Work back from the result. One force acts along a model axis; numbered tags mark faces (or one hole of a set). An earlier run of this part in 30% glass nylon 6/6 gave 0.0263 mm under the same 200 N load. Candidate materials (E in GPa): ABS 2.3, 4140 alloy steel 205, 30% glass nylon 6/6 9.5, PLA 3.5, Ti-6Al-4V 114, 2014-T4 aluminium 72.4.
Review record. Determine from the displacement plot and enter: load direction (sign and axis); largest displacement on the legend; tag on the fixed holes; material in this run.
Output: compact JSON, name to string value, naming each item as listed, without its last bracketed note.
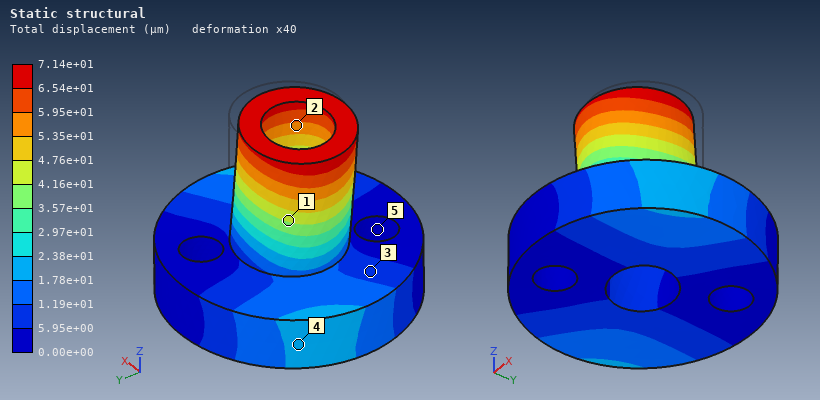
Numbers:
{"load direction": "-X", "largest displacement on the legend": "7.14e+01 µm", "tag on the fixed holes": "5", "material in this run": "PLA"}
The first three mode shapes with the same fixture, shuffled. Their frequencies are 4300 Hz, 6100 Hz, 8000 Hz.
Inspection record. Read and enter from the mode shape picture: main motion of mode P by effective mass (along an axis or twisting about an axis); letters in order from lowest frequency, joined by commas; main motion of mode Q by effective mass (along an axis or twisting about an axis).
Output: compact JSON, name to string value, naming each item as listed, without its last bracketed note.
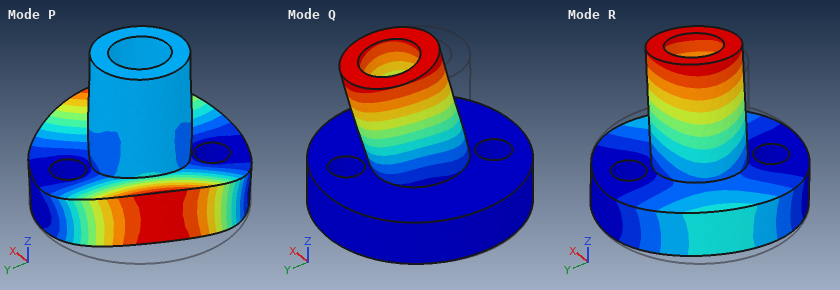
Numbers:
{"main motion of mode P by effective mass": "along Z", "letters in order from lowest frequency, joined by commas": "R, Q, P", "main motion of mode Q by effective mass": "along Y"}
